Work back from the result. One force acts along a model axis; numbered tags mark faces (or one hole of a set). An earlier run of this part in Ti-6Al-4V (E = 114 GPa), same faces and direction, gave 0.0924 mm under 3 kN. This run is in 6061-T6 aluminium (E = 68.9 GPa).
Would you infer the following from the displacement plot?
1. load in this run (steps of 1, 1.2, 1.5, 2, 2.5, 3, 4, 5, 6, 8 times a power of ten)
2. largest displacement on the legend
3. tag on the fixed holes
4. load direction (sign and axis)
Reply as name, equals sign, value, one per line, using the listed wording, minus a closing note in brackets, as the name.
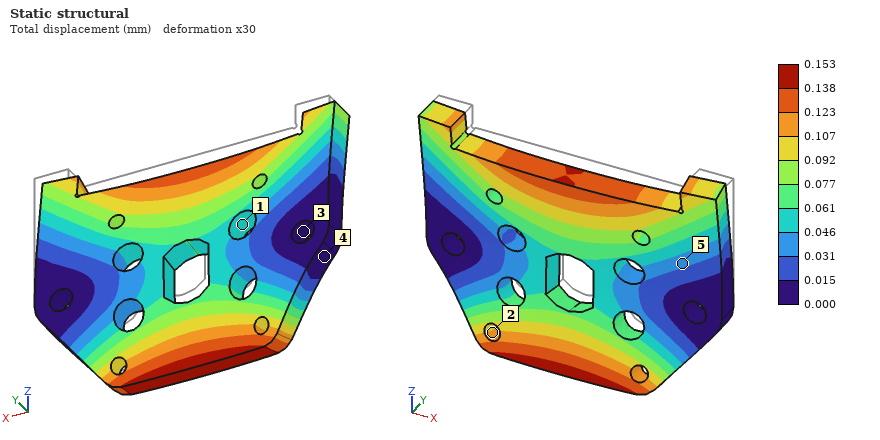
load in this run = 3 kN
largest displacement on the legend = 0.153 mm
tag on the fixed holes = 3
load direction = -Y
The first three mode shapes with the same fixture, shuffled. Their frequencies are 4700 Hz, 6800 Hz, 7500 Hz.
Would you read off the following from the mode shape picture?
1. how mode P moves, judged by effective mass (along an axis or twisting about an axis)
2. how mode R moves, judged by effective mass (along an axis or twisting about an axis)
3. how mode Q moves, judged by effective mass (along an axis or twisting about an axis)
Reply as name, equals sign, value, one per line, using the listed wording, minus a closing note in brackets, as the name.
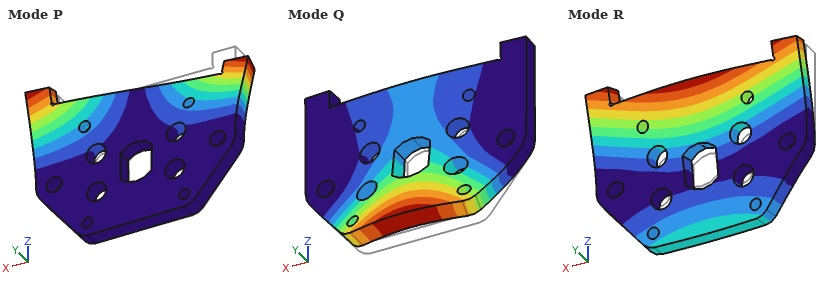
how mode P moves, judged by effective mass = twisting about Z
how mode R moves, judged by effective mass = along Y
how mode Q moves, judged by effective mass = along Y
